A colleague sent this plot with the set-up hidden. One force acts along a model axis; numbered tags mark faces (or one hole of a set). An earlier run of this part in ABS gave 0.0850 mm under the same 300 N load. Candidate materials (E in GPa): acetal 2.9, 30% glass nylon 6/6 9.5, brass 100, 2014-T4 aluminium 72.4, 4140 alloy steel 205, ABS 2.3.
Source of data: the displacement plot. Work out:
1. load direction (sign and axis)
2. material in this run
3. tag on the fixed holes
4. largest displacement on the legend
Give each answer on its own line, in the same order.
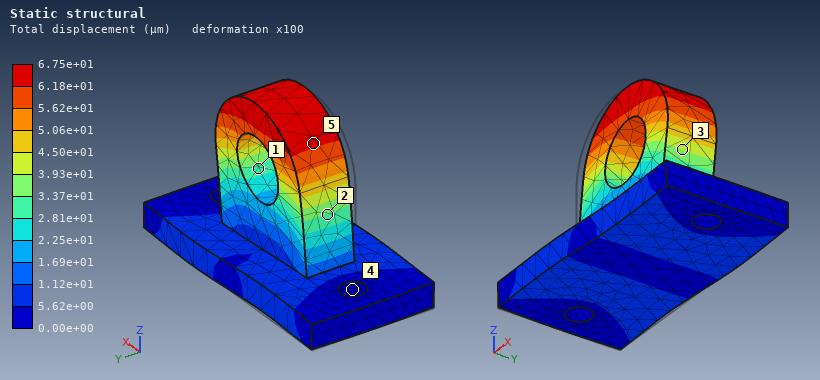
+X
acetal
4
6.75e+01 µm
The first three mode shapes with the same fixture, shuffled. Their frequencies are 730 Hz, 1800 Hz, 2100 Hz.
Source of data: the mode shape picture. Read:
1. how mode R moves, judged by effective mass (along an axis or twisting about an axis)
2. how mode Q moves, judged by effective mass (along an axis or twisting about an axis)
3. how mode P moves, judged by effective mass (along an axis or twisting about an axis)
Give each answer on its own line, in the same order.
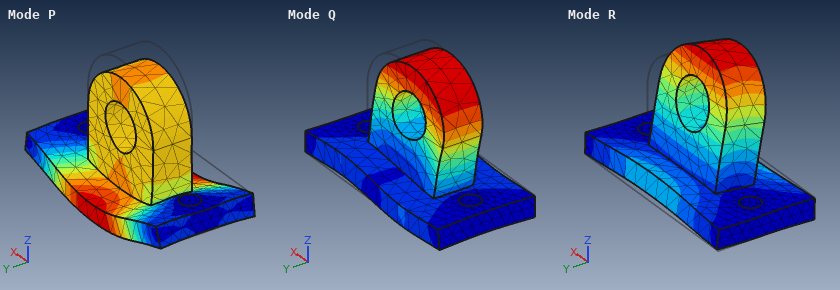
along Y
along X
along Z
